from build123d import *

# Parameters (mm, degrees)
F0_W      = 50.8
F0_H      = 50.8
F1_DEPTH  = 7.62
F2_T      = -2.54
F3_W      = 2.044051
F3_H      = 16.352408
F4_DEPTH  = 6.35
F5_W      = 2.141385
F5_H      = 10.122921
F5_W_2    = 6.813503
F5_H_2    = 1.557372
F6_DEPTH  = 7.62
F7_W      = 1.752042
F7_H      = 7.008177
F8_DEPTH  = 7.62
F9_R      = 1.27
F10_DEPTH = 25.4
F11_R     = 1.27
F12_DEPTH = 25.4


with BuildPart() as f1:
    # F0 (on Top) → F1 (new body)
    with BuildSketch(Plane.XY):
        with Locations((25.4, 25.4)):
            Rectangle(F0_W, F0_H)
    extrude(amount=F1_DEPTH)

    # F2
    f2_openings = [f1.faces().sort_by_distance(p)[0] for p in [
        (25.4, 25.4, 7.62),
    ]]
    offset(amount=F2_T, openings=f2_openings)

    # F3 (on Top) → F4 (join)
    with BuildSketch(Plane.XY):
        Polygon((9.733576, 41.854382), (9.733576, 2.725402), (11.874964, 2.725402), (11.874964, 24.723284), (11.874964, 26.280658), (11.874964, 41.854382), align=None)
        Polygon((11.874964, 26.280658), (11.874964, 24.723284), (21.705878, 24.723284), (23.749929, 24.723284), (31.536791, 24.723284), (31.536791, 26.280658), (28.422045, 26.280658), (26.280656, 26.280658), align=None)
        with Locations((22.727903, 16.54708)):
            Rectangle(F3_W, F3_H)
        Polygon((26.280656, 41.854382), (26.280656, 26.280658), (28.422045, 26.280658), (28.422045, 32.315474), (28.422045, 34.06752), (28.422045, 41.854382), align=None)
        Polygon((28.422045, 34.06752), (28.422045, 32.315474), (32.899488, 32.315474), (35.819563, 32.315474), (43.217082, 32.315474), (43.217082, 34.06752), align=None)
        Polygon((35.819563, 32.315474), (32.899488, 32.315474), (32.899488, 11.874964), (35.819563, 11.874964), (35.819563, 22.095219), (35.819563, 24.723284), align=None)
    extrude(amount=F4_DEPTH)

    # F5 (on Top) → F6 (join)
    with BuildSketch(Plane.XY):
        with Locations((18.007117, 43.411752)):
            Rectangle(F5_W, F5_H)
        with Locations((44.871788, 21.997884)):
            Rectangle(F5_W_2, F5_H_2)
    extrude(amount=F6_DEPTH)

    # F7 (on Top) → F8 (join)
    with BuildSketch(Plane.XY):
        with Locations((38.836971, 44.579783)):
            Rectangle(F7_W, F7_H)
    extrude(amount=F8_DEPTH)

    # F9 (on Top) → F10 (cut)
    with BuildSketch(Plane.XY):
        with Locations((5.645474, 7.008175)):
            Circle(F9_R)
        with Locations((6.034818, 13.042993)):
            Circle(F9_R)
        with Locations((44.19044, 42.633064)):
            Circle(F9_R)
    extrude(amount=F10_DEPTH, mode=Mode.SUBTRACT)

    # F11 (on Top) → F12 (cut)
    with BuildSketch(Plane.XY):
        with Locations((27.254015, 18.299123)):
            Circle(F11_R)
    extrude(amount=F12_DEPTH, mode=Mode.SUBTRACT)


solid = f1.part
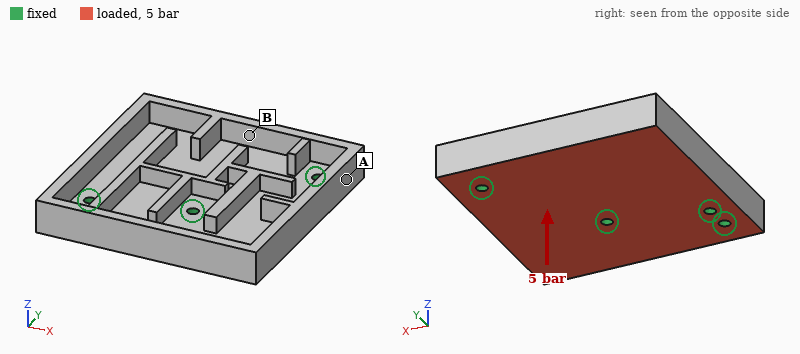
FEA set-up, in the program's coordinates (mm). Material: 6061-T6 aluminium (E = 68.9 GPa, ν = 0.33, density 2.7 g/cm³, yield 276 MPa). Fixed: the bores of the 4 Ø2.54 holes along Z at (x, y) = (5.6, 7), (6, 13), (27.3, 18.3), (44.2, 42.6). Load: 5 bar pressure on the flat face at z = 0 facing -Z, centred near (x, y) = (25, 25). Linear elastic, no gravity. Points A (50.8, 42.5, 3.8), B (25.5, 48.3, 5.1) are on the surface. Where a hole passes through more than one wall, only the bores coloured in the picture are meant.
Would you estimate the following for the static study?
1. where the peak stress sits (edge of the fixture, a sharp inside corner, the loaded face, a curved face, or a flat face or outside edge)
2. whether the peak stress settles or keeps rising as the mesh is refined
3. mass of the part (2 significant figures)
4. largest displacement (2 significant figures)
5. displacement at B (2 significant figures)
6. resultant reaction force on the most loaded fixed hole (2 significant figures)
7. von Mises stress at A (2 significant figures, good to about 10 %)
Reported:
edge of the fixture
keeps rising
28 g
0.17 mm
0.070 mm
620 N
29 MPa
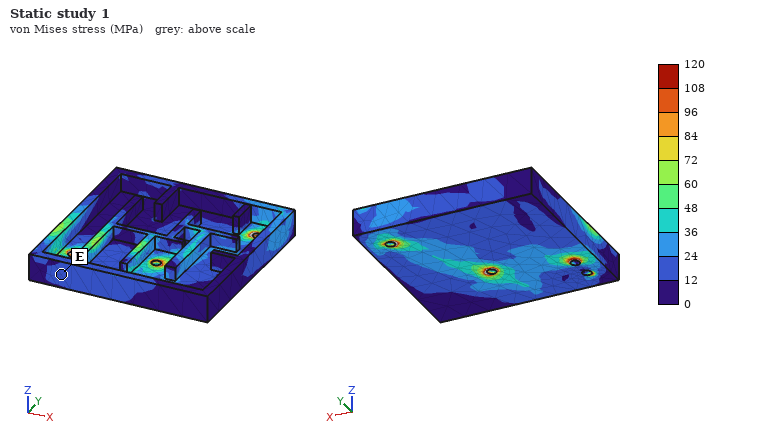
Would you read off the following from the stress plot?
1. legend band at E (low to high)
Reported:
12 to 24 MPa
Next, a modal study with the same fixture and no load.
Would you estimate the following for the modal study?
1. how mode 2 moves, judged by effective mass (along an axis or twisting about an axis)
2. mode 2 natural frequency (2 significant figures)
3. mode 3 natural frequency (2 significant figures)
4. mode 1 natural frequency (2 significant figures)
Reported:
along Z
4000 Hz
10 kHz
3100 Hz
